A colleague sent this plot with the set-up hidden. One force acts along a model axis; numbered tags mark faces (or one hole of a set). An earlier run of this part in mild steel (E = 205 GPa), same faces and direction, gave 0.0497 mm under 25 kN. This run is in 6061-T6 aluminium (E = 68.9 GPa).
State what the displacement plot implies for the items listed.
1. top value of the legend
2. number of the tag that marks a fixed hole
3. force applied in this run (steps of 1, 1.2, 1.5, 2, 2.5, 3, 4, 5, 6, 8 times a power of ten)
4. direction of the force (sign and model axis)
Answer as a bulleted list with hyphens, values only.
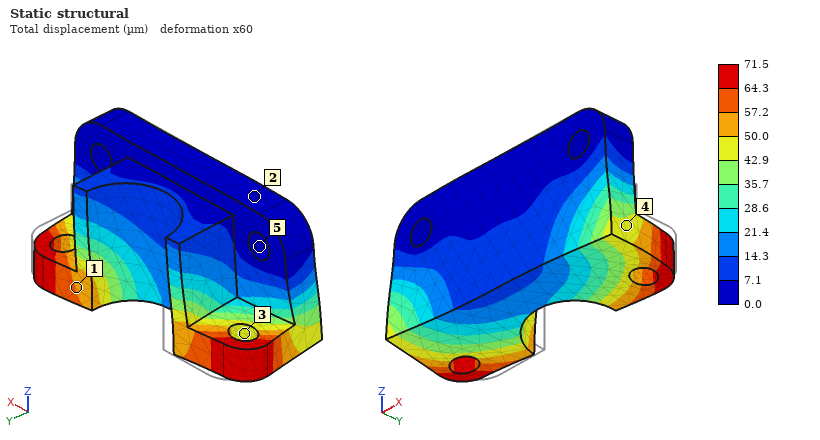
- 71.5 µm
- 5
- 12 kN
- -X
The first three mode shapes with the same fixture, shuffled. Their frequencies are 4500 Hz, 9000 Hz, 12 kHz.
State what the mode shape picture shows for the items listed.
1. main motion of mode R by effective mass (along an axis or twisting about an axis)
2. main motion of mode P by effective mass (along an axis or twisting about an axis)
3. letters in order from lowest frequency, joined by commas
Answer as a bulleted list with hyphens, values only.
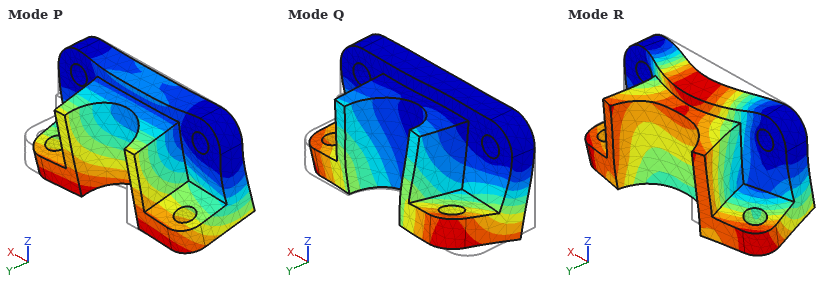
- along Y
- along Y
- P, Q, R
